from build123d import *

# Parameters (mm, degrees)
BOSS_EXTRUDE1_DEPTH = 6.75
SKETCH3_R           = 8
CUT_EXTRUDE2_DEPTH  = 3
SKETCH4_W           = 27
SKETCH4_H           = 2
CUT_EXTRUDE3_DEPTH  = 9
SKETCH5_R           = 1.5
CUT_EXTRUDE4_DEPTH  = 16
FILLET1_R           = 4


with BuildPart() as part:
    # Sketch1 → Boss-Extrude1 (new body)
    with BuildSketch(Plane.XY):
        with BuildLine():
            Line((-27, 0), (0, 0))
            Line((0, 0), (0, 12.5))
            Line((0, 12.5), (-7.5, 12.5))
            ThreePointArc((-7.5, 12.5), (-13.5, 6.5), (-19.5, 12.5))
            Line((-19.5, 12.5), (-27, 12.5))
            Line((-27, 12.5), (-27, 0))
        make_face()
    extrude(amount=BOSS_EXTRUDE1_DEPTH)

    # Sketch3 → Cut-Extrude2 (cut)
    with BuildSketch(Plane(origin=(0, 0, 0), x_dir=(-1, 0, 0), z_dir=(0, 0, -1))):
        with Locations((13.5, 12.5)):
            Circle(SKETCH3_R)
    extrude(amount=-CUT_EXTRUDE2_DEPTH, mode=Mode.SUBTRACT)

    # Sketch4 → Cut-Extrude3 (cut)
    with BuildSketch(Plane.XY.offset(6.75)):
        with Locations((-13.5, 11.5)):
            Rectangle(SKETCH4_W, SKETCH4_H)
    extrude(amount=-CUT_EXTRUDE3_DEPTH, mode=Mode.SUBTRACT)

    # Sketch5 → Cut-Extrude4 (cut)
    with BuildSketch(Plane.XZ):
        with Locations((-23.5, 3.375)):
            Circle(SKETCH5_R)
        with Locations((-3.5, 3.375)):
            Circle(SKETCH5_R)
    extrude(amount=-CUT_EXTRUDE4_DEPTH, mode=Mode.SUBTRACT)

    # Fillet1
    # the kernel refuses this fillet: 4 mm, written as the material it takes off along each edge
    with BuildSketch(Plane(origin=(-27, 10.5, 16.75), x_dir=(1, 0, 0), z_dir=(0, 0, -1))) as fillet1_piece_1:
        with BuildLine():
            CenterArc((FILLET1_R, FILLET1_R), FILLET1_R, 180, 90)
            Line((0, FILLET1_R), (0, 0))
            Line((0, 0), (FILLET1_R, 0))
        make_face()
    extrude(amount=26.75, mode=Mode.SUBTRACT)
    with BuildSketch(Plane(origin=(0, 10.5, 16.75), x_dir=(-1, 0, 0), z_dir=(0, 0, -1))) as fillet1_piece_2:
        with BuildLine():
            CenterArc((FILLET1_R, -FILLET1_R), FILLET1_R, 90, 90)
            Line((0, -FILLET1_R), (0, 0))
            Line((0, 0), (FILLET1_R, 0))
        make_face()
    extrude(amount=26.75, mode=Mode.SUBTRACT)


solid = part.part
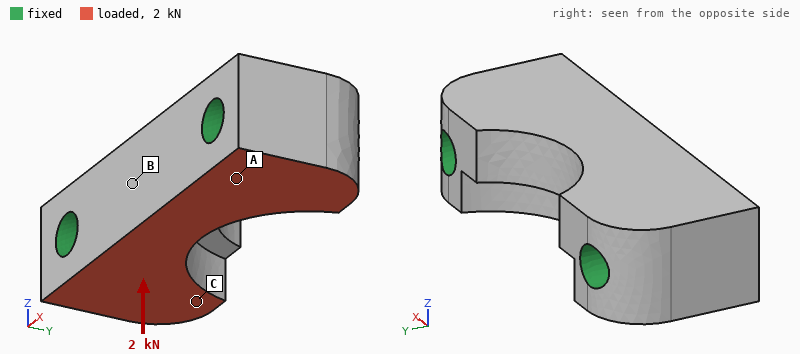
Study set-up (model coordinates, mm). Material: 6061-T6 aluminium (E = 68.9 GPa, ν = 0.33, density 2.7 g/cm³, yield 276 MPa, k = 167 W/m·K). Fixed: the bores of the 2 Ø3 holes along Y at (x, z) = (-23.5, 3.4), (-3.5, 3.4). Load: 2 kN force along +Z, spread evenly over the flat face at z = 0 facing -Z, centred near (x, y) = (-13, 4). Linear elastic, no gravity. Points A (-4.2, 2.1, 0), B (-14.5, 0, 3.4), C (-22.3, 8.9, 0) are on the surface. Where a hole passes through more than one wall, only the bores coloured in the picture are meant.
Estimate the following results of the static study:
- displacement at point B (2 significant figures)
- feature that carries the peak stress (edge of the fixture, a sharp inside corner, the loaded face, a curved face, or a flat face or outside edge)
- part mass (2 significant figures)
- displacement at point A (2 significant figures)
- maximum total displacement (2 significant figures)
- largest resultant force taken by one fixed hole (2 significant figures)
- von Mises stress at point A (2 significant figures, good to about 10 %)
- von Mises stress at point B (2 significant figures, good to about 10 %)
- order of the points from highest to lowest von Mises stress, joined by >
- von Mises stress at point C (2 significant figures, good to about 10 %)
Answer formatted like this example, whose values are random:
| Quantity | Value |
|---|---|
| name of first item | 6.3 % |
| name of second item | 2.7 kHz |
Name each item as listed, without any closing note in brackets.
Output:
| Quantity | Value |
|---|---|
| displacement at point B | 4.8 µm |
| feature that carries the peak stress | edge of the fixture |
| part mass | 3.8 g |
| displacement at point A | 0.87 µm |
| maximum total displacement | 5.3 µm |
| largest resultant force taken by one fixed hole | 1.0 kN |
| von Mises stress at point A | 26 MPa |
| von Mises stress at point B | 6.3 MPa |
| order of the points from highest to lowest von Mises stress, joined by > | A > C > B |
| von Mises stress at point C | 16 MPa |
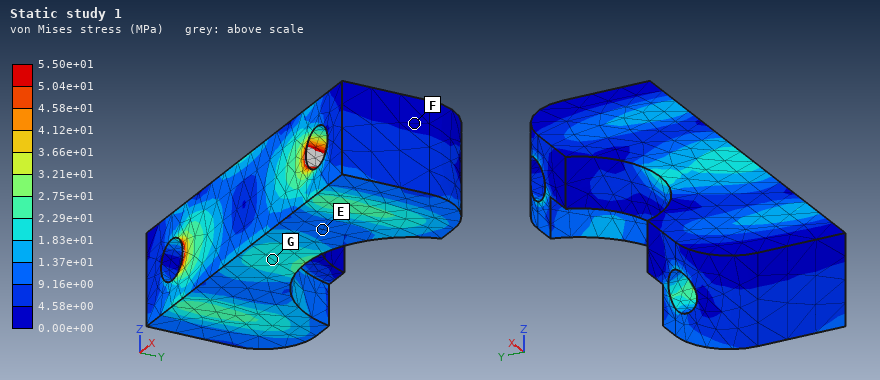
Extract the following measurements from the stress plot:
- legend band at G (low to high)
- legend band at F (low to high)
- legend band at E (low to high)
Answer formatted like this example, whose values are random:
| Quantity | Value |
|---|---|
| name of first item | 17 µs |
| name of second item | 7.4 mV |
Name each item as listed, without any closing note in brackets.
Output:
| Quantity | Value |
|---|---|
| legend band at G | 1.83e+01 to 2.29e+01 MPa |
| legend band at F | 0.00e+00 to 4.58e+00 MPa |
| legend band at E | 9.16e+00 to 1.37e+01 MPa |
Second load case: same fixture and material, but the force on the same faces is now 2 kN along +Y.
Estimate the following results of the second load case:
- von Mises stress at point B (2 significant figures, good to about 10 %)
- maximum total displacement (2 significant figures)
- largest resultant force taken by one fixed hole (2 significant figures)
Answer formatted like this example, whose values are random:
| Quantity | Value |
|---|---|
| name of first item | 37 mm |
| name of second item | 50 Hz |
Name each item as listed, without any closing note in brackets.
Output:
| Quantity | Value |
|---|---|
| von Mises stress at point B | 18 MPa |
| maximum total displacement | 7.7 µm |
| largest resultant force taken by one fixed hole | 1.0 kN |
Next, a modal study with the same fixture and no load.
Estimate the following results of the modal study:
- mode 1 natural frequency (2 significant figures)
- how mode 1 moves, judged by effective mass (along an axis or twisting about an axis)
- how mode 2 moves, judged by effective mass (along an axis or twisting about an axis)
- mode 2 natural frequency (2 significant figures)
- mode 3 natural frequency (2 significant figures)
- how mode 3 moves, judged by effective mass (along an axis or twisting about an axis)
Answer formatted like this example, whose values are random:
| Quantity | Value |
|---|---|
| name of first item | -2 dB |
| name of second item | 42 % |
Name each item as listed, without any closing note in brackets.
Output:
| Quantity | Value |
|---|---|
| mode 1 natural frequency | 59 kHz |
| how mode 1 moves, judged by effective mass | along Z |
| how mode 2 moves, judged by effective mass | along Y |
| mode 2 natural frequency | 78 kHz |
| mode 3 natural frequency | 96 kHz |
| how mode 3 moves, judged by effective mass | twisting about X |
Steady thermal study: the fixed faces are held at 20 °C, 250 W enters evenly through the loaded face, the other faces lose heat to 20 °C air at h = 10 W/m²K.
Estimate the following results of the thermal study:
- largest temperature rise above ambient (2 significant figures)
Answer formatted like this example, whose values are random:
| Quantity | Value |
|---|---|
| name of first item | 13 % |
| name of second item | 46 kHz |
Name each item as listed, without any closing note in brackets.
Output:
| Quantity | Value |
|---|---|
| largest temperature rise above ambient | 52 K |
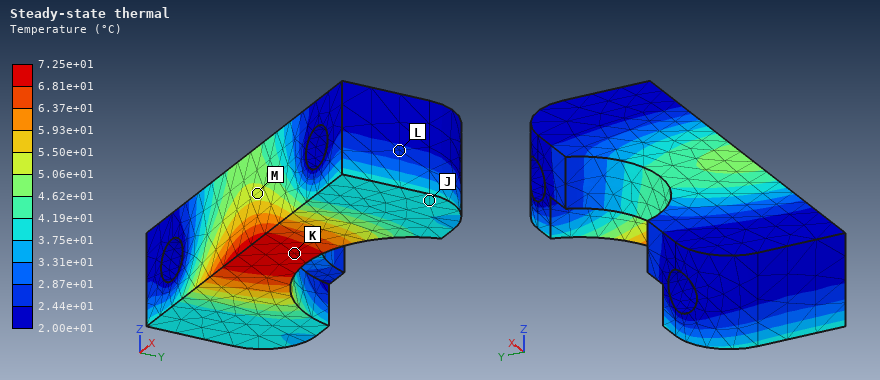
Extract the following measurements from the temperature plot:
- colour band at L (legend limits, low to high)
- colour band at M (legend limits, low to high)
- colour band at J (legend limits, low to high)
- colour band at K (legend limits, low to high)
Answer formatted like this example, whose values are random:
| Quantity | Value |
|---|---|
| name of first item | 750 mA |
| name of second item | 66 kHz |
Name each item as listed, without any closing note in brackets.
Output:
| Quantity | Value |
|---|---|
| colour band at L | 2.44e+01 to 2.87e+01 °C |
| colour band at M | 5.06e+01 to 5.50e+01 °C |
| colour band at J | 3.75e+01 to 4.19e+01 °C |
| colour band at K | 6.81e+01 to 7.25e+01 °C |
